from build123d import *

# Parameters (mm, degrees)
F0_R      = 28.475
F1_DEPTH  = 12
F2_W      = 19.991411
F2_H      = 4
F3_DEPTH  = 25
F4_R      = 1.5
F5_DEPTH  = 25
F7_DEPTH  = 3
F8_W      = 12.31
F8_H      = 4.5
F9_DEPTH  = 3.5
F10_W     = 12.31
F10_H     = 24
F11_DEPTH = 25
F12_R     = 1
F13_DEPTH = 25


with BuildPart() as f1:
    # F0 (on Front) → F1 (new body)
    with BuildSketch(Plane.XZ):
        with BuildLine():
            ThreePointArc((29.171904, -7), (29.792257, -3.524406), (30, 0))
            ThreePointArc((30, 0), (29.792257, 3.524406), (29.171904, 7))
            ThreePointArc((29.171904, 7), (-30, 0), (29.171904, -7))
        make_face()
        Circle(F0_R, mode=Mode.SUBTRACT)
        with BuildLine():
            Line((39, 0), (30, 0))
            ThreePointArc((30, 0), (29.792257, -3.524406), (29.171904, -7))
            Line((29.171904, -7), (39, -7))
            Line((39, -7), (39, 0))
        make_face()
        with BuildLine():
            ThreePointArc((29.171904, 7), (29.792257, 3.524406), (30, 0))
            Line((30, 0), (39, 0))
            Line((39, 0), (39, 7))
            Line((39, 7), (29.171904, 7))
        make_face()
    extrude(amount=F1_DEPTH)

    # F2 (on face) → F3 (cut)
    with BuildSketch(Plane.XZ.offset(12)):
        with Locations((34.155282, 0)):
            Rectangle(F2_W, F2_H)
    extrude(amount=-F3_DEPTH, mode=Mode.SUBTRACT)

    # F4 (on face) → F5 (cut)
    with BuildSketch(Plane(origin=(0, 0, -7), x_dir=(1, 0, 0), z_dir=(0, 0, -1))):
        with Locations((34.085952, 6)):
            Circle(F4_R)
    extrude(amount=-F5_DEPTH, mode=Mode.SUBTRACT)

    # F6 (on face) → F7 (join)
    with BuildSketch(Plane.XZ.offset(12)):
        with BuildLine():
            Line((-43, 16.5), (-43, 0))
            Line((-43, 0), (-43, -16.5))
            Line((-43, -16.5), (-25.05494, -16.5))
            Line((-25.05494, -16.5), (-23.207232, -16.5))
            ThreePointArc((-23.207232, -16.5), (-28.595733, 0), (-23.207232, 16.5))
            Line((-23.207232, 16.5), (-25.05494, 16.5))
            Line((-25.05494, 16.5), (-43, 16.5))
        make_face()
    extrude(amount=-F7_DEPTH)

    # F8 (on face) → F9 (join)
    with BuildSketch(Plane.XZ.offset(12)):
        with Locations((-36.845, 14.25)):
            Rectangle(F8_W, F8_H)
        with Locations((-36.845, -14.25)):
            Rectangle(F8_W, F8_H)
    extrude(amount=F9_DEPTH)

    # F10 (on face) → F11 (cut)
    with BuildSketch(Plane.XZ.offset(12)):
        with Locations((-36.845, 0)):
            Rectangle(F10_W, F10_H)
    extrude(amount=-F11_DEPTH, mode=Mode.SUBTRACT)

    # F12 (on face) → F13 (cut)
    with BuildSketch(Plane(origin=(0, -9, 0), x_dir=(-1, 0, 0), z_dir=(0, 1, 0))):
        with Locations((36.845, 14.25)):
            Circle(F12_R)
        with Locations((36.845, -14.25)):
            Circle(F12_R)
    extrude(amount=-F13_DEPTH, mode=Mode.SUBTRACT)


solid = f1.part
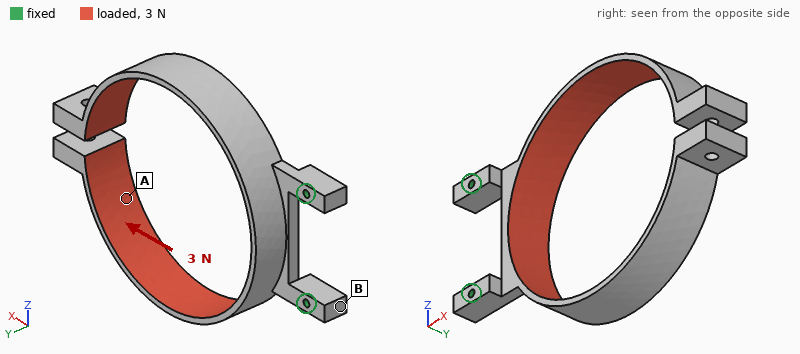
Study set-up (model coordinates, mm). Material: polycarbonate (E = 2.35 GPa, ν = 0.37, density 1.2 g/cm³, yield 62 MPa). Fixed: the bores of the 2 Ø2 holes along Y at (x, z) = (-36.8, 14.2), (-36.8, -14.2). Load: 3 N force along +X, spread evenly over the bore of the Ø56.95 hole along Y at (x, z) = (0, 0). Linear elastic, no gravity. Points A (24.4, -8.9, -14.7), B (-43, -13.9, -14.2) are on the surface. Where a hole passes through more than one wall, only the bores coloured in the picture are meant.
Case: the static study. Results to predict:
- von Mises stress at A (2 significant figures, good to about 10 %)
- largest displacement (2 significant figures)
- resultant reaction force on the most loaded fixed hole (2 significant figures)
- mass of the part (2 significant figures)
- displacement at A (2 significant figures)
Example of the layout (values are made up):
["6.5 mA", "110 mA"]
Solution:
["0.36 MPa", "1.1 mm", "1.7 N", "6.3 g", "0.60 mm"]
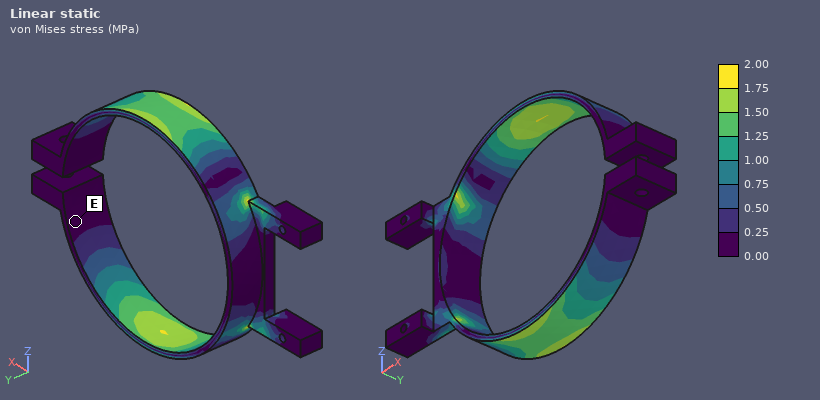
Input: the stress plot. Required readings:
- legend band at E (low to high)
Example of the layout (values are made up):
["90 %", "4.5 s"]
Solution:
["0.00 to 0.25 MPa"]
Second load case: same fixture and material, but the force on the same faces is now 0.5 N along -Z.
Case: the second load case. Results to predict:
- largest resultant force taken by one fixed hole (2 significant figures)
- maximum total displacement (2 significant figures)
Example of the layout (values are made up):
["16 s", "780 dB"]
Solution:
["0.42 N", "1.1 mm"]
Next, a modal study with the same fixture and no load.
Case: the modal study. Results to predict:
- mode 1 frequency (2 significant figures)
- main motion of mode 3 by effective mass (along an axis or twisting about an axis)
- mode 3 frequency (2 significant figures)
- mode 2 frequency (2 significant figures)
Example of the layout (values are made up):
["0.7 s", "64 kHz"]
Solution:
["43 Hz", "along Y", "62 Hz", "43 Hz"]
